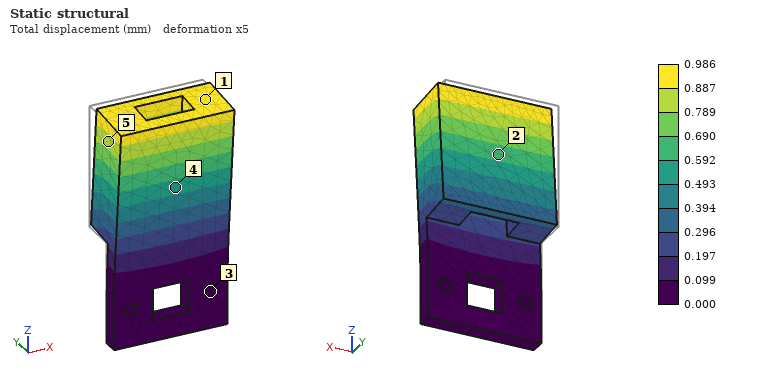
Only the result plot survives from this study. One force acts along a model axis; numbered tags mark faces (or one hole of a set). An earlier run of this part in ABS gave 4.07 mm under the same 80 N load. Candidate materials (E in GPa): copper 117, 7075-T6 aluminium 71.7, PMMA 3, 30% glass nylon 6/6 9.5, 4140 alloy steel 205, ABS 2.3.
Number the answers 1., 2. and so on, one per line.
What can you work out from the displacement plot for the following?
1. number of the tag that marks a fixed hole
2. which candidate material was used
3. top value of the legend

1. 3
2. 30% glass nylon 6/6
3. 0.986 mm
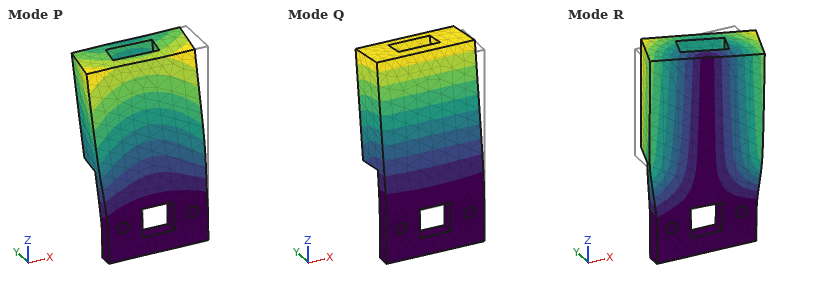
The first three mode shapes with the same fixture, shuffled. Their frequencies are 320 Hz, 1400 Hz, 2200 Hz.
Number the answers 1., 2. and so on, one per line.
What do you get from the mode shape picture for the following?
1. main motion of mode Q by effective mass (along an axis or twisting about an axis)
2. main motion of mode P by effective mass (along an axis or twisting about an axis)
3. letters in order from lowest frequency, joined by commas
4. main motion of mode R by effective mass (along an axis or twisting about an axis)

1. along Y
2. along X
3. Q, R, P
4. along X
